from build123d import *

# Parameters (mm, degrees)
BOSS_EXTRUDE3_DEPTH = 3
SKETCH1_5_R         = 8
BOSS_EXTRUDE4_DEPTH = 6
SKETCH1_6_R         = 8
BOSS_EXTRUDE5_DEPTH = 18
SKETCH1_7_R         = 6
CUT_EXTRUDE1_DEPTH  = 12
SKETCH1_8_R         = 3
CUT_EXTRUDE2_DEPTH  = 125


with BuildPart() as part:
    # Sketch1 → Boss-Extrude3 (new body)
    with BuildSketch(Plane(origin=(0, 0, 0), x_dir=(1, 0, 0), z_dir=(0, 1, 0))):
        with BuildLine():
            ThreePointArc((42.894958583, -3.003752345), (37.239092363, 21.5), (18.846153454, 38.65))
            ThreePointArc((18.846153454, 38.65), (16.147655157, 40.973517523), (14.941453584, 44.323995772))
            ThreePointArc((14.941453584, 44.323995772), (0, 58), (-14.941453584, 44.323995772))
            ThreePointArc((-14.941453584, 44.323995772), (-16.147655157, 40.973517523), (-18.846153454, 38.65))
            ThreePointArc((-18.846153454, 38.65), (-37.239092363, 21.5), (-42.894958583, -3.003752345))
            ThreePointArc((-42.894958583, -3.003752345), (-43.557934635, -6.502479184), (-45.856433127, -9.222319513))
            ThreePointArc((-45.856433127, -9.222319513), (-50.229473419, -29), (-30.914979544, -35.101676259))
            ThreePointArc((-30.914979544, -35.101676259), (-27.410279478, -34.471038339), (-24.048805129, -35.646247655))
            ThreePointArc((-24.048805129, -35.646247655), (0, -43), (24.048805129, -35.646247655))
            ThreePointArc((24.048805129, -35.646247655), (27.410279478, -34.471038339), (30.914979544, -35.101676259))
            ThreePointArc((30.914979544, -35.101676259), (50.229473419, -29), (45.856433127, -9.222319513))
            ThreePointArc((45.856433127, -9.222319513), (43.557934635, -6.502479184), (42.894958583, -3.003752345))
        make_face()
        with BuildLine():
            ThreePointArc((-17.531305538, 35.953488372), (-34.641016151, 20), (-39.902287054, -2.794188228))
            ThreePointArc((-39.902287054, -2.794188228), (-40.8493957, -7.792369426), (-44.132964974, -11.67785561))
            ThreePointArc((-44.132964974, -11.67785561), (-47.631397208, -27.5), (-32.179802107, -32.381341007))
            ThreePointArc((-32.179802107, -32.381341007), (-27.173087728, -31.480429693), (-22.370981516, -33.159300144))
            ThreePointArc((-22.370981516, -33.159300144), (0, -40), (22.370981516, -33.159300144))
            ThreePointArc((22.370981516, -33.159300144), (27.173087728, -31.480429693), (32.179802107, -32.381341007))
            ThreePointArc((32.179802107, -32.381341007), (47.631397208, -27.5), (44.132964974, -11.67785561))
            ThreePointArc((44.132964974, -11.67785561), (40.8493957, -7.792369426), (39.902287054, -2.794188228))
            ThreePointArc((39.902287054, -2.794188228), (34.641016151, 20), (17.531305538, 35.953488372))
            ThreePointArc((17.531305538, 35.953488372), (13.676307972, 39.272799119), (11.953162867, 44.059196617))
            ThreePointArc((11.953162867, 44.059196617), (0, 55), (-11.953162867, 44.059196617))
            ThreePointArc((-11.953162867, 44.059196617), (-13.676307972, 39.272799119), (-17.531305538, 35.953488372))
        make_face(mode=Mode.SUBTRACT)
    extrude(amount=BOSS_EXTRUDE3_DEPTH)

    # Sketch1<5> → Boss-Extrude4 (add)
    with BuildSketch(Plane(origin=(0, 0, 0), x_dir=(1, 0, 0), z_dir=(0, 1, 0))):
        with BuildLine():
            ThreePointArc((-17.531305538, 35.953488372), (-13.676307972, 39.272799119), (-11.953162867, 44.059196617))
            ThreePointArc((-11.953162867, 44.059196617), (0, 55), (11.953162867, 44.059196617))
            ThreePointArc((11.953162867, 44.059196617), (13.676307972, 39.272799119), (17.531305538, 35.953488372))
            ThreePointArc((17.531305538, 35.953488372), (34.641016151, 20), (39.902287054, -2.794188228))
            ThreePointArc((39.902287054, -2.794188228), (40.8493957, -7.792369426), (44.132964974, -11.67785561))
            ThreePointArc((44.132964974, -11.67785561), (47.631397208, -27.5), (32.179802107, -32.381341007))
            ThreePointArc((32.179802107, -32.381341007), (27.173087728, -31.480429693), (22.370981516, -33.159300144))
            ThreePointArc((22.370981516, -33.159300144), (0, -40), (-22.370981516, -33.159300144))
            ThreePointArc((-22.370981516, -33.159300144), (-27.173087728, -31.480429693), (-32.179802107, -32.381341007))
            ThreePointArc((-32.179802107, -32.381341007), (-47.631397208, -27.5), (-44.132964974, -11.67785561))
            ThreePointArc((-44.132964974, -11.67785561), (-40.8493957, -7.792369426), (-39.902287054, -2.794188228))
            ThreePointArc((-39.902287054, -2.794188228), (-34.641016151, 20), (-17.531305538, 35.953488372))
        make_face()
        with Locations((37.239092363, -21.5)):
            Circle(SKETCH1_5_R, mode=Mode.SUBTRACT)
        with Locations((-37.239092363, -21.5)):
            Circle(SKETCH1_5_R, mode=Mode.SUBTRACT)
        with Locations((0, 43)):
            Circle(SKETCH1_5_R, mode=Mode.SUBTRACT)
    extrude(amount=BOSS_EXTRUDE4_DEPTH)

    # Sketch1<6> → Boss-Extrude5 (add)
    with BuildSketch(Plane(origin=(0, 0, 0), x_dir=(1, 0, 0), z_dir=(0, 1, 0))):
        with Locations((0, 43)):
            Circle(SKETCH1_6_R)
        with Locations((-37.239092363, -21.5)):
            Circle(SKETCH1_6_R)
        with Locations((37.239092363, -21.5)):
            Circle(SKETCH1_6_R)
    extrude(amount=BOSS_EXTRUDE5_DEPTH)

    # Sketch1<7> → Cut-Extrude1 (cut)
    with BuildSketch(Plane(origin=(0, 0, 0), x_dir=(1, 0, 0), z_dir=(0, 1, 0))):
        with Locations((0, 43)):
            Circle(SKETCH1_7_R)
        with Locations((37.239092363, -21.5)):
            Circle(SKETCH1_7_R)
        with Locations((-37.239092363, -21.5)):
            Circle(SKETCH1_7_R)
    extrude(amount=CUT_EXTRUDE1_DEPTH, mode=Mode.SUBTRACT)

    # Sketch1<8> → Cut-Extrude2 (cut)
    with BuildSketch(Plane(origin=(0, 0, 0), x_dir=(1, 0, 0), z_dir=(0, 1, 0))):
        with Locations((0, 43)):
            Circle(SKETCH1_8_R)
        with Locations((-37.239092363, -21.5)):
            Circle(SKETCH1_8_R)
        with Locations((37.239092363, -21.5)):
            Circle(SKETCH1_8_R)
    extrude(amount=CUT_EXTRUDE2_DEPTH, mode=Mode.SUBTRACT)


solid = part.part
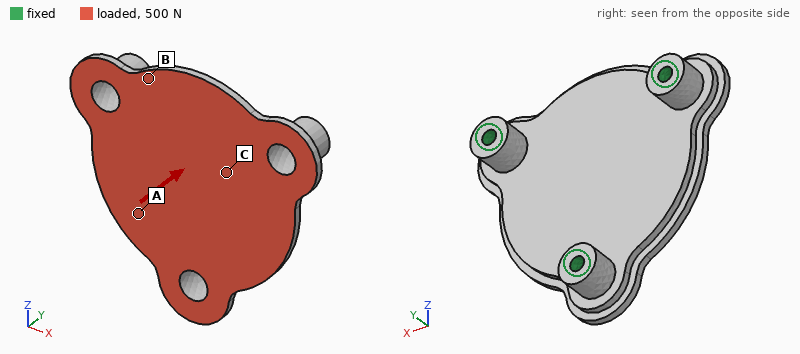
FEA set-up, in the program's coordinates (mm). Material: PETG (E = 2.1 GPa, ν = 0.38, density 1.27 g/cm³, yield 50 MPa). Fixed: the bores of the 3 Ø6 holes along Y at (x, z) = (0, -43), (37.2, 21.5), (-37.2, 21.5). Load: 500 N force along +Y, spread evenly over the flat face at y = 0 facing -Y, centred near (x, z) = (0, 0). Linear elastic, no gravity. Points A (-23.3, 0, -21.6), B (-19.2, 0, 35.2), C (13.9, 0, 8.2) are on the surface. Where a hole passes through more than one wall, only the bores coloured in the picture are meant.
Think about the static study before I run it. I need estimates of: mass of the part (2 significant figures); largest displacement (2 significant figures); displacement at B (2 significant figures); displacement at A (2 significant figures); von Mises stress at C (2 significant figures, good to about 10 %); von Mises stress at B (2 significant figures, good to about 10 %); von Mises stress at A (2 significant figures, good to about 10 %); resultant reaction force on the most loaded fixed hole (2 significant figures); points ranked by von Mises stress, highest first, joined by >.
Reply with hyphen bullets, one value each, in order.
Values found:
- 53 g
- 0.25 mm
- 0.14 mm
- 0.20 mm
- 2.5 MPa
- 1.5 MPa
- 3.2 MPa
- 190 N
- A > C > B
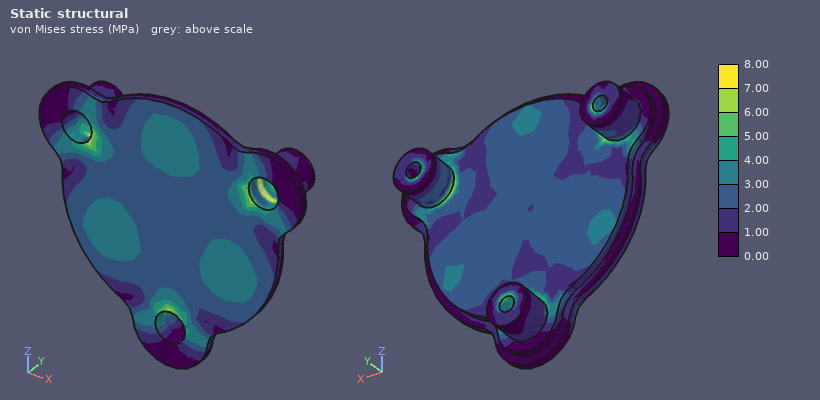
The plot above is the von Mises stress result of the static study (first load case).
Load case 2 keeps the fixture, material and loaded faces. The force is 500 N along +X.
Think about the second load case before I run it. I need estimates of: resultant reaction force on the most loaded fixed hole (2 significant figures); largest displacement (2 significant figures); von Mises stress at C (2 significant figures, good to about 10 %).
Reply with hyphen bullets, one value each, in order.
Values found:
- 180 N
- 0.16 mm
- 1.4 MPa
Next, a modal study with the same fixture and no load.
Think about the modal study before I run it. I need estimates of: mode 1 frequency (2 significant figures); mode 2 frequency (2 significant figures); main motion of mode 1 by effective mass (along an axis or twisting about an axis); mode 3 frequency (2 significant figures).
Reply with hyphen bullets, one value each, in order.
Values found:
- 1200 Hz
- 1200 Hz
- along Y
- 1200 Hz
